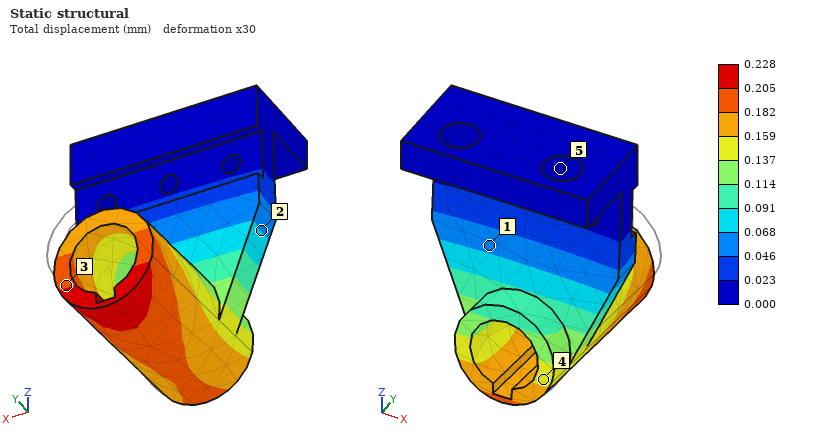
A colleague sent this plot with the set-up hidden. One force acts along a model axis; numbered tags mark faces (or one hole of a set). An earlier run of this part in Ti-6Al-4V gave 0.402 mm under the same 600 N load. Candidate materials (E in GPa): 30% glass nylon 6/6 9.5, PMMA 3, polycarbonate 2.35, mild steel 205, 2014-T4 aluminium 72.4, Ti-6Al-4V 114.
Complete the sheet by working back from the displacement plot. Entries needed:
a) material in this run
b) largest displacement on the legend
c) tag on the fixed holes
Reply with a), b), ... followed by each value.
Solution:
a) mild steel
b) 0.228 mm
c) 5
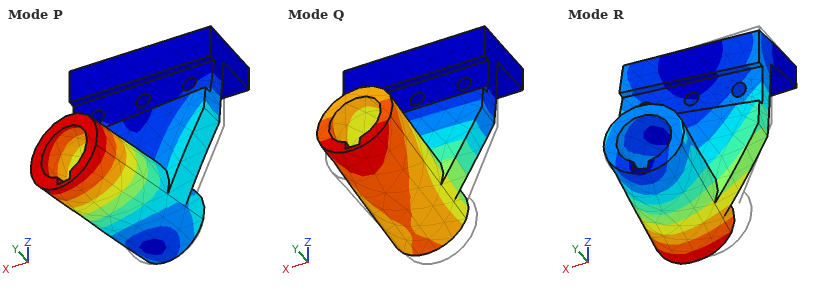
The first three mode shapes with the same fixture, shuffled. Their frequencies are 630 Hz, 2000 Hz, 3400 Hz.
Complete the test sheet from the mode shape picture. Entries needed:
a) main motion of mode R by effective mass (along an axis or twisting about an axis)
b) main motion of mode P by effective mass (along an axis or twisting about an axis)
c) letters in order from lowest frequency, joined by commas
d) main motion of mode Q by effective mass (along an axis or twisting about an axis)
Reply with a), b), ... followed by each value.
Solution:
a) along X
b) along X
c) Q, P, R
d) along Y
